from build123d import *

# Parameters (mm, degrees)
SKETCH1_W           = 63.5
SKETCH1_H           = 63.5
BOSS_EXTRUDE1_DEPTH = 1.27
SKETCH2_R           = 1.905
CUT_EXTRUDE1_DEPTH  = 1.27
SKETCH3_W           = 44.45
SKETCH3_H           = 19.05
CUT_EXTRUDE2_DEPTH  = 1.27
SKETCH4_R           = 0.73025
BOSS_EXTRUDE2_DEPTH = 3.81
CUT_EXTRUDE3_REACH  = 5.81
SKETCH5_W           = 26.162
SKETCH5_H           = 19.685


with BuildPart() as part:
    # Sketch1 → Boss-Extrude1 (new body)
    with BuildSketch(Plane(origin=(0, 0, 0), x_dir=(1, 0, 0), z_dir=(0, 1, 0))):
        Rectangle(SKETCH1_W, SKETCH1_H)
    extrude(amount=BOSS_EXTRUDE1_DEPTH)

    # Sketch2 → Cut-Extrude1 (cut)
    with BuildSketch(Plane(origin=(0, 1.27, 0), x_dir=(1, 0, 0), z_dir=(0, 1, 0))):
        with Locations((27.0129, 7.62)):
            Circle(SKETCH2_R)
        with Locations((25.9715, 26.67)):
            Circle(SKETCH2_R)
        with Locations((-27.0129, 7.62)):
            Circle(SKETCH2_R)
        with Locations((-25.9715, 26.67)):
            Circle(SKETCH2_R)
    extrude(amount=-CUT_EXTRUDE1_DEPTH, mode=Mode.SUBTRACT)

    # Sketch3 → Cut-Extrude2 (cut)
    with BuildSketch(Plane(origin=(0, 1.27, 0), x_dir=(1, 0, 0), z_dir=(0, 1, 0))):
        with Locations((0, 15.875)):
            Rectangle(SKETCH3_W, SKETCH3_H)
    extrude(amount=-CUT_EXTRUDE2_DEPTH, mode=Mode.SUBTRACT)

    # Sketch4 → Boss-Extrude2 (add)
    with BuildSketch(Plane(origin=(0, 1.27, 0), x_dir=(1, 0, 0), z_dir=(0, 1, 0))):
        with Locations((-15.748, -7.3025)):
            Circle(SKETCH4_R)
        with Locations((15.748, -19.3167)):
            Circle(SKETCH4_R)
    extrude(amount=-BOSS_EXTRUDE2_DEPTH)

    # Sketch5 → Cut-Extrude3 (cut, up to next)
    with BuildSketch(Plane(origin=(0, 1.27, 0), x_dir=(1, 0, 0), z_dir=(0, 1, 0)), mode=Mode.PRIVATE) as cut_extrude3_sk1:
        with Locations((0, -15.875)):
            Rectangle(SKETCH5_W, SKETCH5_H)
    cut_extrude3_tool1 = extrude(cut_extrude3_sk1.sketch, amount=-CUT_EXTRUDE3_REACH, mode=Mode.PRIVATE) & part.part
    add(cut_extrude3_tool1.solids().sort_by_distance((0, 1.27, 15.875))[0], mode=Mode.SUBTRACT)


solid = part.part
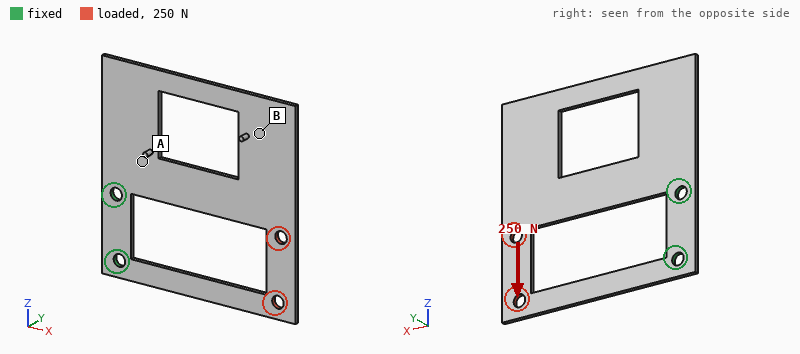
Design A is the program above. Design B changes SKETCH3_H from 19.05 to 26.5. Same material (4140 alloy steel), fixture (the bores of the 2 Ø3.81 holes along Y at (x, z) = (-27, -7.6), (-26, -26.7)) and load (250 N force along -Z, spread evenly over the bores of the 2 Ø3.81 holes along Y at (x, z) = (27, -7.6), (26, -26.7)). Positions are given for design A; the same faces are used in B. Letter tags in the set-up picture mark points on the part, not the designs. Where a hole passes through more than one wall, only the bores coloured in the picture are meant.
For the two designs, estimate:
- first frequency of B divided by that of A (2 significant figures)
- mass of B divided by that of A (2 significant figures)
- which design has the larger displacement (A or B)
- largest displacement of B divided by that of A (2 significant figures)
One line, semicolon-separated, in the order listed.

0.85; 0.87; B; 1.9
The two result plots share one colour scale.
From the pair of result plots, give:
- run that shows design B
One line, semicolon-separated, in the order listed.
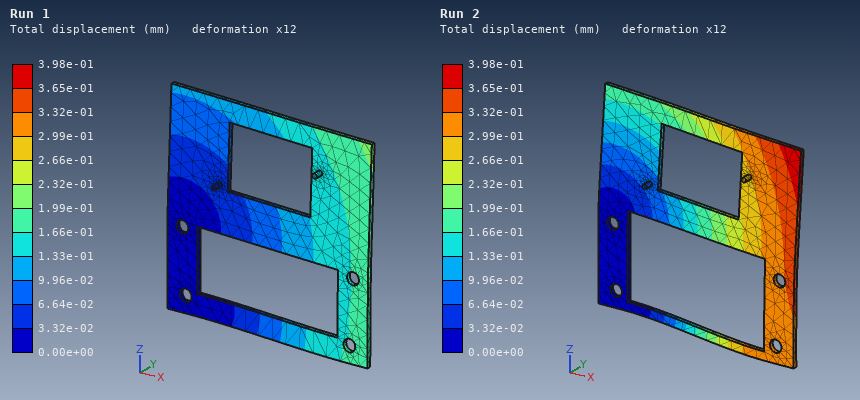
Run 2
